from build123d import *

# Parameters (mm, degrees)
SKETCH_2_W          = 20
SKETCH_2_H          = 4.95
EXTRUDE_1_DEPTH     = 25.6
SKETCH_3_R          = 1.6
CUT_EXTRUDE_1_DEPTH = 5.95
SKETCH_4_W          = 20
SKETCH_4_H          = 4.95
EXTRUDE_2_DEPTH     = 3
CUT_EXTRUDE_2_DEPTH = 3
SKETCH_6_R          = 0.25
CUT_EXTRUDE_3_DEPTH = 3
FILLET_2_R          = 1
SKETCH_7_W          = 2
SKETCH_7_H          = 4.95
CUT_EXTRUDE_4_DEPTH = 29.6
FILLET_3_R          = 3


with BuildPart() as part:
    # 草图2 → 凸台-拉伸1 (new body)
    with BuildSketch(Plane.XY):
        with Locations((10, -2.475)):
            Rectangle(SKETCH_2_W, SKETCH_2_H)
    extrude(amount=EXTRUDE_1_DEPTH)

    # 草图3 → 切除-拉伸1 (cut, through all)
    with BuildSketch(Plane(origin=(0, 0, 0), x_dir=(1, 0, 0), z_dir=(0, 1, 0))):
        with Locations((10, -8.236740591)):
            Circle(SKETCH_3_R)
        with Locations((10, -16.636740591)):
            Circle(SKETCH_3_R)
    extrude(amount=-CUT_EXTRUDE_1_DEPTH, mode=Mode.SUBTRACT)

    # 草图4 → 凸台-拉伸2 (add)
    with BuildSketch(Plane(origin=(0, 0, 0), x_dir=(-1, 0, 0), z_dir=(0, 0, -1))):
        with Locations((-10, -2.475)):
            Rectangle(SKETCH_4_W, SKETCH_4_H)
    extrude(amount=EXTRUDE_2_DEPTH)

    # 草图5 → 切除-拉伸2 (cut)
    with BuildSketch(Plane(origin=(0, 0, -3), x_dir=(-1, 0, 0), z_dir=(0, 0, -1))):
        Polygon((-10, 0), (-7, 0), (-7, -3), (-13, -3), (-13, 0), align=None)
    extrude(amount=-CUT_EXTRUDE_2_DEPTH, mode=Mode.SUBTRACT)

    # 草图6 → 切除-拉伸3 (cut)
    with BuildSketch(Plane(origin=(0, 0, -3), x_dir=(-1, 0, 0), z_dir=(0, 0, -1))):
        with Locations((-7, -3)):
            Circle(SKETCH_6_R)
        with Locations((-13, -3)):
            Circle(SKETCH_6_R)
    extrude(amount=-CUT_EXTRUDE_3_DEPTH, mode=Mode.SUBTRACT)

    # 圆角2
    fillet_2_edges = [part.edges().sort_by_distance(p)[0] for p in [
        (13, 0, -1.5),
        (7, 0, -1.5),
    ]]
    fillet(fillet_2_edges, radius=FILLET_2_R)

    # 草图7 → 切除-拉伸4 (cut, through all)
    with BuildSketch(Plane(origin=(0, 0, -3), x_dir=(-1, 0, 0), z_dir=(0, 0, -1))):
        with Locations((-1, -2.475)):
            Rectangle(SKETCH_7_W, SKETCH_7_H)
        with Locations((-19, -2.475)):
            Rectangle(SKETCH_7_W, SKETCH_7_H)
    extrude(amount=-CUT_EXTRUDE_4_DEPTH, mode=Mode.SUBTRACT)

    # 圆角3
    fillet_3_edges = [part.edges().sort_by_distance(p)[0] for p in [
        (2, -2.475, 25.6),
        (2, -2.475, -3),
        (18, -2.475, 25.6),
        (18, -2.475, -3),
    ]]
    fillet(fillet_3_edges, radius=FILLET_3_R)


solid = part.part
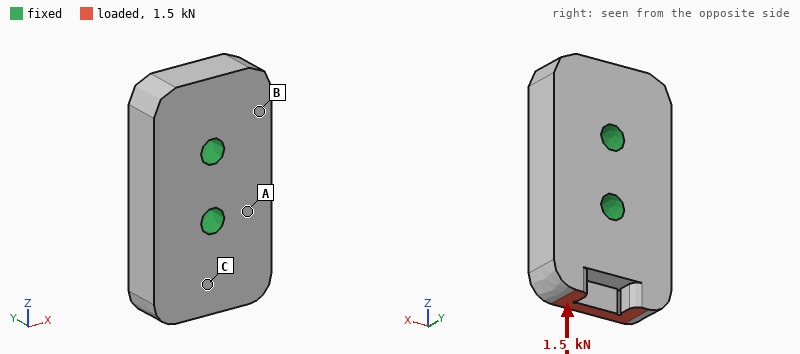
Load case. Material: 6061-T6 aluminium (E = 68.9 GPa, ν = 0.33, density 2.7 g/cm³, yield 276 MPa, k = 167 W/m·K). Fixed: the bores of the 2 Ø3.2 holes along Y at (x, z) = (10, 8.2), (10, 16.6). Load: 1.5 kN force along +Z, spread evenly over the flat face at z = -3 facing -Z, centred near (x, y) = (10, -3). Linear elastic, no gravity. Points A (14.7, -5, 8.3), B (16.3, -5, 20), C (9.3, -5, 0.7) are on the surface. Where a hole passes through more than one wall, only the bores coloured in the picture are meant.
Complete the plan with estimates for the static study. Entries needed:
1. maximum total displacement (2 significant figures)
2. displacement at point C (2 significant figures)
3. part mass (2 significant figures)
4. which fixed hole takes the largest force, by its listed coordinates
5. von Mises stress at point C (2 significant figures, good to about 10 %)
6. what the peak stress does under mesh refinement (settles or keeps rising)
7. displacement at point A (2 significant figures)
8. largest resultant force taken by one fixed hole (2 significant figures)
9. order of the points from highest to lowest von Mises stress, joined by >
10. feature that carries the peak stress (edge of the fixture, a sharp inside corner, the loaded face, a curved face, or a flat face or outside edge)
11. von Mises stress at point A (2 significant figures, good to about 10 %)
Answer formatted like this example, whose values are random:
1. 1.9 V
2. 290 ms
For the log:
1. 9.7 µm
2. 5.8 µm
3. 5.6 g
4. (10, 8.2)
5. 53 MPa
6. keeps rising
7. 1.5 µm
8. 1.2 kN
9. C > A > B
10. a sharp inside corner
11. 19 MPa
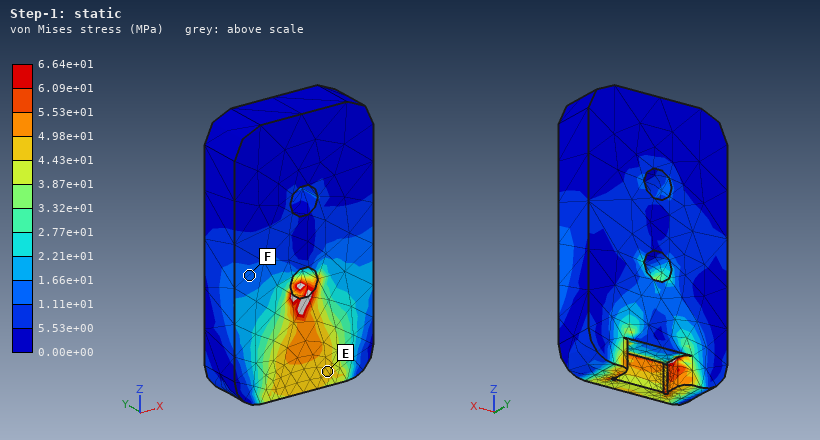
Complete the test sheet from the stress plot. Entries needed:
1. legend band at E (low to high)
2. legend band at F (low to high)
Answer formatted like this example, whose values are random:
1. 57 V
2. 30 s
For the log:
1. 4.43e+01 to 4.98e+01 MPa
2. 1.11e+01 to 1.66e+01 MPa
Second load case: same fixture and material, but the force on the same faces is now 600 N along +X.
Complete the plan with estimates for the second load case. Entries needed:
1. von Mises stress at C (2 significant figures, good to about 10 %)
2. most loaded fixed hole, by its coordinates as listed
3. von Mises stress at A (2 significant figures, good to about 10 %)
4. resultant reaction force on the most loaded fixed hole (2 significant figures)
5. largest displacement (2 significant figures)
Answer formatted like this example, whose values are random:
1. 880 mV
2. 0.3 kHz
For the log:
1. 25 MPa
2. (10, 8.2)
3. 18 MPa
4. 1.1 kN
5. 13 µm
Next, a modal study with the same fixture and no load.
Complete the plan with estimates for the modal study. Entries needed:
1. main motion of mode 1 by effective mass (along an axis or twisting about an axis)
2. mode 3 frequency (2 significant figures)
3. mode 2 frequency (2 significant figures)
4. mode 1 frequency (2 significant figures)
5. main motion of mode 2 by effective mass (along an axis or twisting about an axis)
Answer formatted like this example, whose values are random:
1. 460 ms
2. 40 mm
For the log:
1. along Y
2. 38 kHz
3. 35 kHz
4. 30 kHz
5. twisting about Z
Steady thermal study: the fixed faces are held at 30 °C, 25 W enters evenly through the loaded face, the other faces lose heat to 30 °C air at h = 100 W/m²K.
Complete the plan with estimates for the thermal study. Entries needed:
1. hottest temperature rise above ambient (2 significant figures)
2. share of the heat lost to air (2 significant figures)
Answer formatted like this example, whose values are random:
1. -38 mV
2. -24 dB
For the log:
1. 32 K
2. 3.0 %
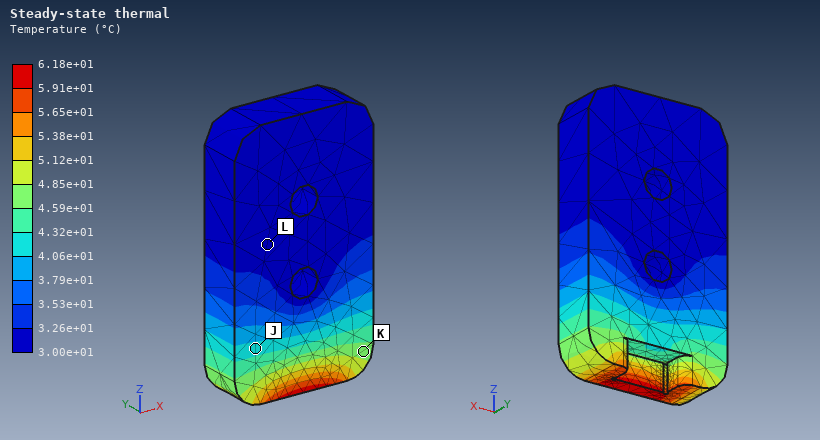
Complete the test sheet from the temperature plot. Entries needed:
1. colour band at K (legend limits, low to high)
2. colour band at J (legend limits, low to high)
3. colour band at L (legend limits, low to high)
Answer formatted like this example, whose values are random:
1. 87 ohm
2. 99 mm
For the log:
1. 4.59e+01 to 4.85e+01 °C
2. 4.06e+01 to 4.32e+01 °C
3. 3.00e+01 to 3.26e+01 °C
